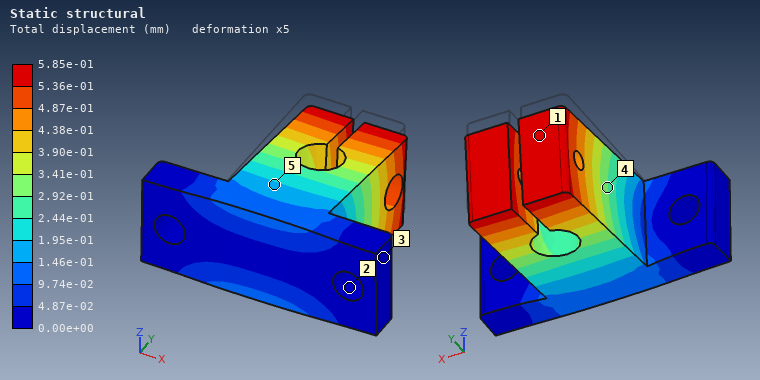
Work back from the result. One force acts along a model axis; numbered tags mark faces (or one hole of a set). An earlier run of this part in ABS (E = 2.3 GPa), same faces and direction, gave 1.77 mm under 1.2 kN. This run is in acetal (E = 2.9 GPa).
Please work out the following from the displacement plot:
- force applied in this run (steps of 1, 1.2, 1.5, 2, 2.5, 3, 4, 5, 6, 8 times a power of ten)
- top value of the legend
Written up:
500 N
5.85e-01 mm
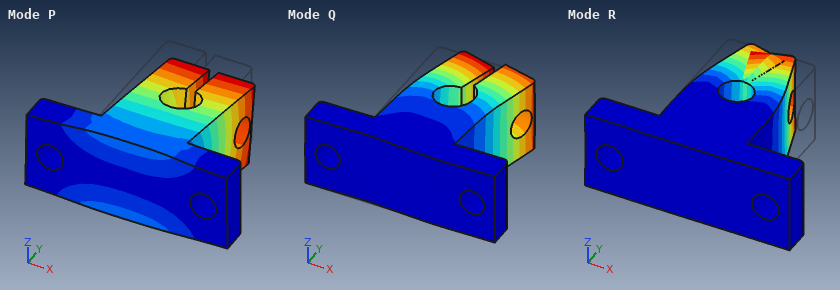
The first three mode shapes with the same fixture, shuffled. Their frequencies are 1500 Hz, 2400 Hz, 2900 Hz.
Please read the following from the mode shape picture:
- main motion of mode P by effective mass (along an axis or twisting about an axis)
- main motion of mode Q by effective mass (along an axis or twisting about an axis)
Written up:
along Z
along X
